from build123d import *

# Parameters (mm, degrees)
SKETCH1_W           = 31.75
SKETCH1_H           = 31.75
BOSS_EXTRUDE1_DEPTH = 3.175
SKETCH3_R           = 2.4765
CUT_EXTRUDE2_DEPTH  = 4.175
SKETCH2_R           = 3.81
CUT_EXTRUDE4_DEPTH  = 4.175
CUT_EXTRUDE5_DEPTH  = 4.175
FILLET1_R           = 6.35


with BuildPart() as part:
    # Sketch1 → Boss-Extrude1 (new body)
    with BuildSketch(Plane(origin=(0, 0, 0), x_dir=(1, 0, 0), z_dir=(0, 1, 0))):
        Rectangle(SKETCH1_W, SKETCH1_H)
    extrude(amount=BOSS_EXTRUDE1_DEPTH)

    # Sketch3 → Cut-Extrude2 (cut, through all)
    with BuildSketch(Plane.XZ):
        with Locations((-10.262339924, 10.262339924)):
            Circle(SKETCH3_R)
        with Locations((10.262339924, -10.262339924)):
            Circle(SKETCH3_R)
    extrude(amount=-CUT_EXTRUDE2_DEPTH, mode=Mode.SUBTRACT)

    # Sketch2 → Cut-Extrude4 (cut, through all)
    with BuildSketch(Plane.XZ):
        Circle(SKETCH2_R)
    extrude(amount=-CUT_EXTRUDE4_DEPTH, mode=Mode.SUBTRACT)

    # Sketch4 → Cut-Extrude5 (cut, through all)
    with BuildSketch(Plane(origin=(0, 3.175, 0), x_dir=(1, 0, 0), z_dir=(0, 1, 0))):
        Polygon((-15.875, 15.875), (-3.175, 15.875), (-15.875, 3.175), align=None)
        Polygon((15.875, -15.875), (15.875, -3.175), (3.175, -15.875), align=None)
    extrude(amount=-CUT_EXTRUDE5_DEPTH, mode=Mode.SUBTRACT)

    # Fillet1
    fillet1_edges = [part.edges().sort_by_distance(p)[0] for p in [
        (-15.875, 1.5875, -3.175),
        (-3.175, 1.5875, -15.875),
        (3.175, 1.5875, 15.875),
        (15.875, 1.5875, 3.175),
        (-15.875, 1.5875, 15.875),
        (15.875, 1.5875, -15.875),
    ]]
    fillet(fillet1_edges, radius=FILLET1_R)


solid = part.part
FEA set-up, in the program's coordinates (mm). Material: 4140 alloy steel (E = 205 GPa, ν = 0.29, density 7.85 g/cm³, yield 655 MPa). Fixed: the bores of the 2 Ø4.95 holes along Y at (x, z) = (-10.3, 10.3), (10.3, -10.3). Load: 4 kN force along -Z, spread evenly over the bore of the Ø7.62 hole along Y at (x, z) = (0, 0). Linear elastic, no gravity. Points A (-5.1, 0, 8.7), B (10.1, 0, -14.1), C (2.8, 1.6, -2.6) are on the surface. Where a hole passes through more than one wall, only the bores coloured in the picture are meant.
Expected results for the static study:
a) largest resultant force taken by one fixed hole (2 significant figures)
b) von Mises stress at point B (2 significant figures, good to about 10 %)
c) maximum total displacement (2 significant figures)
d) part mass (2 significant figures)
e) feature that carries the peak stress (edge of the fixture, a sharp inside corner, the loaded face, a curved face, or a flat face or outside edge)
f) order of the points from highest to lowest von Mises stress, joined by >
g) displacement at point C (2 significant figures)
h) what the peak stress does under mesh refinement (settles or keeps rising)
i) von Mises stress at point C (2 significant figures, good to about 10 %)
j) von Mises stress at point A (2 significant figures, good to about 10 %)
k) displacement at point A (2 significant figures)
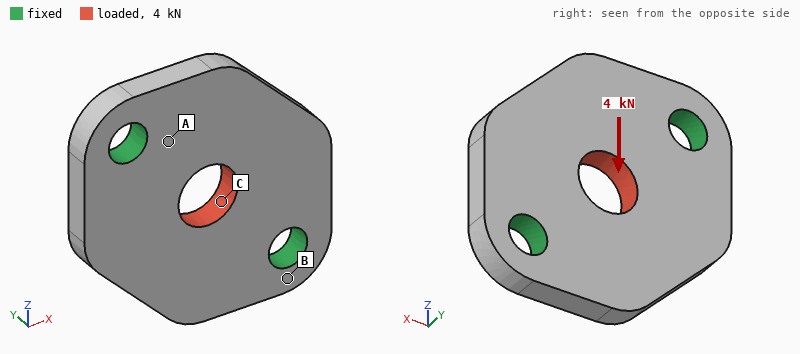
2.0 kN
18 MPa
5.0 µm
18 g
edge of the fixture
C > A > B
4.3 µm
keeps rising
79 MPa
53 MPa
2.0 µm
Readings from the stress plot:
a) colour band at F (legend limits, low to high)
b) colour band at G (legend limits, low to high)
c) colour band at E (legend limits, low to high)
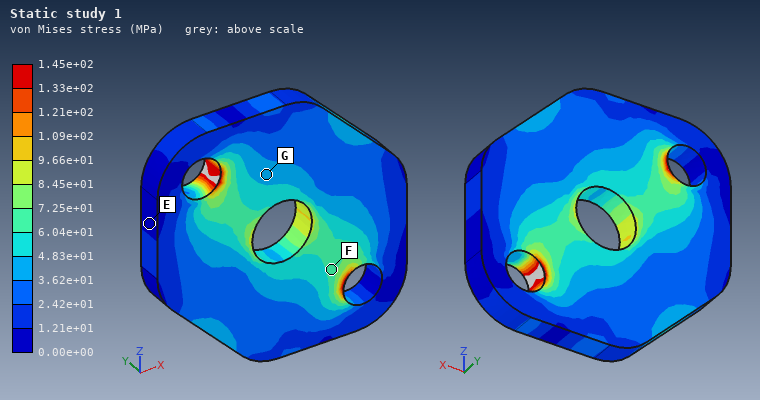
6.04e+01 to 7.25e+01 MPa
3.62e+01 to 4.83e+01 MPa
0.00e+00 to 1.21e+01 MPa
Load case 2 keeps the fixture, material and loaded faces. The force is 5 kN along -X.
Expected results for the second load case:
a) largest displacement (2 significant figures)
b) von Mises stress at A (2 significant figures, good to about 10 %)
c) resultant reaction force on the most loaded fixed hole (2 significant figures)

6.2 µm
83 MPa
2.5 kN
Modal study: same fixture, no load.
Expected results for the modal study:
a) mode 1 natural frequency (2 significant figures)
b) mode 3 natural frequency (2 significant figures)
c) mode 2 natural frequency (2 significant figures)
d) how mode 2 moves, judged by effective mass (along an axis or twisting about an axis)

12 kHz
29 kHz
14 kHz
along Y
